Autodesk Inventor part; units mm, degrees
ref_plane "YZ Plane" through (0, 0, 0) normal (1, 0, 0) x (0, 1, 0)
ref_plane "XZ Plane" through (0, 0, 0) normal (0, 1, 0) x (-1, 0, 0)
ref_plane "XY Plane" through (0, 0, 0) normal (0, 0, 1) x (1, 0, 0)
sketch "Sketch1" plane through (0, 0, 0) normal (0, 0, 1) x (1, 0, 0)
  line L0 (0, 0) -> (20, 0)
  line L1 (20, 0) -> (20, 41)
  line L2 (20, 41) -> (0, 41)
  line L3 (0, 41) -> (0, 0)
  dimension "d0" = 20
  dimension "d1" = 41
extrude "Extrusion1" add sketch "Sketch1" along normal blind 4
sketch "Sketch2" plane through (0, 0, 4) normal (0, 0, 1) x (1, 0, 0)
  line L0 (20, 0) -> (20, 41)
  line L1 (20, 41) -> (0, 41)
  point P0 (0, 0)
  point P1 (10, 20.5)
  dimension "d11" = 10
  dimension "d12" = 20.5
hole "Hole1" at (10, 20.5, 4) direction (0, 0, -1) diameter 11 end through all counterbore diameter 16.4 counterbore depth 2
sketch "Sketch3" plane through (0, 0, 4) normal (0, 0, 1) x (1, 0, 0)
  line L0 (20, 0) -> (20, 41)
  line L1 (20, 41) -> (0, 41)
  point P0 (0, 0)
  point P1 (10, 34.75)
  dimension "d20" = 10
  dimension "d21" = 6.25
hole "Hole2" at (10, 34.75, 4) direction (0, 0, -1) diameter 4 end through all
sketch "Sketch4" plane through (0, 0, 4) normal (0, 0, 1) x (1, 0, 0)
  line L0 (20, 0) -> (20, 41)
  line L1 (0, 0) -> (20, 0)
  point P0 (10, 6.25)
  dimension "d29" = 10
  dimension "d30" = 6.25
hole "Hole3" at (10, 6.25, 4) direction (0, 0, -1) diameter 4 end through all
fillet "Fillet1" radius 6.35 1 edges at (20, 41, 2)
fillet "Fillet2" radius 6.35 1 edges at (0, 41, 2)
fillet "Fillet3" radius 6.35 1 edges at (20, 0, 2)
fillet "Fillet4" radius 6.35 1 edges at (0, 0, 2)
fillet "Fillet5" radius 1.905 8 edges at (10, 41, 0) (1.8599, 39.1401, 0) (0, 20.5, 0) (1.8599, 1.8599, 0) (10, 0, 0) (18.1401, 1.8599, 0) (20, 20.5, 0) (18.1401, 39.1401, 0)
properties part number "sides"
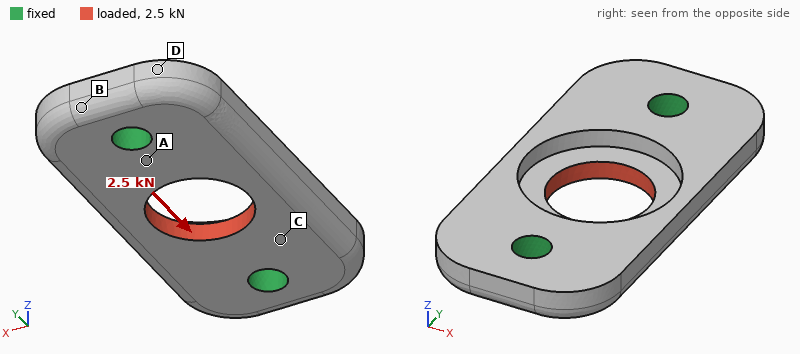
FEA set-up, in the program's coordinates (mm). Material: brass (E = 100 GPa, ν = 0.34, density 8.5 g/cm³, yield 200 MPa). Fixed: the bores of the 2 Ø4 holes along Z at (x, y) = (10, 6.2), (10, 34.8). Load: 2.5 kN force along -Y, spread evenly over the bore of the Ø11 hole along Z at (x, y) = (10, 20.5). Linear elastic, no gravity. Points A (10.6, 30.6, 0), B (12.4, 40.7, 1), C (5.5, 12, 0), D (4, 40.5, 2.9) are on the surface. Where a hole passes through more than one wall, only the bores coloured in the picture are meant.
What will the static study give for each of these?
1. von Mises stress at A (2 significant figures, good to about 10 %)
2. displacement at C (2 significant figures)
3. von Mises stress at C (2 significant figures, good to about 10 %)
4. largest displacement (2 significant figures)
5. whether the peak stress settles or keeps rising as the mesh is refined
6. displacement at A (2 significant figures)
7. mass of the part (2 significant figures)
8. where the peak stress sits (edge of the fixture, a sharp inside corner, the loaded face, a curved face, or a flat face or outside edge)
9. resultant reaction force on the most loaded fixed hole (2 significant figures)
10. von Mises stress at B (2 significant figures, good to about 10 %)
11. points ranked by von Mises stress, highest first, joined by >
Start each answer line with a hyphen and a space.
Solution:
- 56 MPa
- 2.9 µm
- 35 MPa
- 5.6 µm
- keeps rising
- 1.4 µm
- 20 g
- edge of the fixture
- 1.3 kN
- 14 MPa
- A > C > B > D
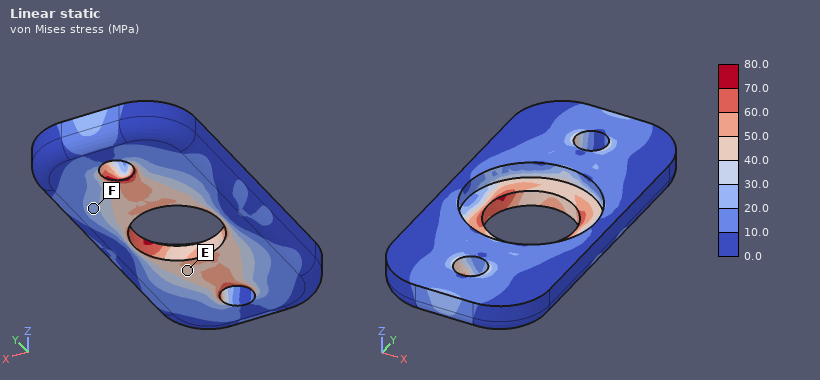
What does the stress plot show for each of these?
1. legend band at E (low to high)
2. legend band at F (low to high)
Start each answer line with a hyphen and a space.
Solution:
- 40.0 to 50.0 MPa
- 20.0 to 30.0 MPa
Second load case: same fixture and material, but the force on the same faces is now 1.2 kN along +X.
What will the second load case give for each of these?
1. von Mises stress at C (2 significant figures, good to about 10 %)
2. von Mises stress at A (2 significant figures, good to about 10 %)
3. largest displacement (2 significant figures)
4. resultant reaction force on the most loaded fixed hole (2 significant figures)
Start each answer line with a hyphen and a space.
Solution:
- 23 MPa
- 27 MPa
- 6.9 µm
- 600 N
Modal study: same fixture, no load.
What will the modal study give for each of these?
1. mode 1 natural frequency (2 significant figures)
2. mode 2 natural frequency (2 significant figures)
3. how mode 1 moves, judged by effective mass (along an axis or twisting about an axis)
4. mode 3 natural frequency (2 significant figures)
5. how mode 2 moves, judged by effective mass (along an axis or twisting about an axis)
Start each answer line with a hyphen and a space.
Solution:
- 14 kHz
- 15 kHz
- twisting about Y
- 23 kHz
- along Z
